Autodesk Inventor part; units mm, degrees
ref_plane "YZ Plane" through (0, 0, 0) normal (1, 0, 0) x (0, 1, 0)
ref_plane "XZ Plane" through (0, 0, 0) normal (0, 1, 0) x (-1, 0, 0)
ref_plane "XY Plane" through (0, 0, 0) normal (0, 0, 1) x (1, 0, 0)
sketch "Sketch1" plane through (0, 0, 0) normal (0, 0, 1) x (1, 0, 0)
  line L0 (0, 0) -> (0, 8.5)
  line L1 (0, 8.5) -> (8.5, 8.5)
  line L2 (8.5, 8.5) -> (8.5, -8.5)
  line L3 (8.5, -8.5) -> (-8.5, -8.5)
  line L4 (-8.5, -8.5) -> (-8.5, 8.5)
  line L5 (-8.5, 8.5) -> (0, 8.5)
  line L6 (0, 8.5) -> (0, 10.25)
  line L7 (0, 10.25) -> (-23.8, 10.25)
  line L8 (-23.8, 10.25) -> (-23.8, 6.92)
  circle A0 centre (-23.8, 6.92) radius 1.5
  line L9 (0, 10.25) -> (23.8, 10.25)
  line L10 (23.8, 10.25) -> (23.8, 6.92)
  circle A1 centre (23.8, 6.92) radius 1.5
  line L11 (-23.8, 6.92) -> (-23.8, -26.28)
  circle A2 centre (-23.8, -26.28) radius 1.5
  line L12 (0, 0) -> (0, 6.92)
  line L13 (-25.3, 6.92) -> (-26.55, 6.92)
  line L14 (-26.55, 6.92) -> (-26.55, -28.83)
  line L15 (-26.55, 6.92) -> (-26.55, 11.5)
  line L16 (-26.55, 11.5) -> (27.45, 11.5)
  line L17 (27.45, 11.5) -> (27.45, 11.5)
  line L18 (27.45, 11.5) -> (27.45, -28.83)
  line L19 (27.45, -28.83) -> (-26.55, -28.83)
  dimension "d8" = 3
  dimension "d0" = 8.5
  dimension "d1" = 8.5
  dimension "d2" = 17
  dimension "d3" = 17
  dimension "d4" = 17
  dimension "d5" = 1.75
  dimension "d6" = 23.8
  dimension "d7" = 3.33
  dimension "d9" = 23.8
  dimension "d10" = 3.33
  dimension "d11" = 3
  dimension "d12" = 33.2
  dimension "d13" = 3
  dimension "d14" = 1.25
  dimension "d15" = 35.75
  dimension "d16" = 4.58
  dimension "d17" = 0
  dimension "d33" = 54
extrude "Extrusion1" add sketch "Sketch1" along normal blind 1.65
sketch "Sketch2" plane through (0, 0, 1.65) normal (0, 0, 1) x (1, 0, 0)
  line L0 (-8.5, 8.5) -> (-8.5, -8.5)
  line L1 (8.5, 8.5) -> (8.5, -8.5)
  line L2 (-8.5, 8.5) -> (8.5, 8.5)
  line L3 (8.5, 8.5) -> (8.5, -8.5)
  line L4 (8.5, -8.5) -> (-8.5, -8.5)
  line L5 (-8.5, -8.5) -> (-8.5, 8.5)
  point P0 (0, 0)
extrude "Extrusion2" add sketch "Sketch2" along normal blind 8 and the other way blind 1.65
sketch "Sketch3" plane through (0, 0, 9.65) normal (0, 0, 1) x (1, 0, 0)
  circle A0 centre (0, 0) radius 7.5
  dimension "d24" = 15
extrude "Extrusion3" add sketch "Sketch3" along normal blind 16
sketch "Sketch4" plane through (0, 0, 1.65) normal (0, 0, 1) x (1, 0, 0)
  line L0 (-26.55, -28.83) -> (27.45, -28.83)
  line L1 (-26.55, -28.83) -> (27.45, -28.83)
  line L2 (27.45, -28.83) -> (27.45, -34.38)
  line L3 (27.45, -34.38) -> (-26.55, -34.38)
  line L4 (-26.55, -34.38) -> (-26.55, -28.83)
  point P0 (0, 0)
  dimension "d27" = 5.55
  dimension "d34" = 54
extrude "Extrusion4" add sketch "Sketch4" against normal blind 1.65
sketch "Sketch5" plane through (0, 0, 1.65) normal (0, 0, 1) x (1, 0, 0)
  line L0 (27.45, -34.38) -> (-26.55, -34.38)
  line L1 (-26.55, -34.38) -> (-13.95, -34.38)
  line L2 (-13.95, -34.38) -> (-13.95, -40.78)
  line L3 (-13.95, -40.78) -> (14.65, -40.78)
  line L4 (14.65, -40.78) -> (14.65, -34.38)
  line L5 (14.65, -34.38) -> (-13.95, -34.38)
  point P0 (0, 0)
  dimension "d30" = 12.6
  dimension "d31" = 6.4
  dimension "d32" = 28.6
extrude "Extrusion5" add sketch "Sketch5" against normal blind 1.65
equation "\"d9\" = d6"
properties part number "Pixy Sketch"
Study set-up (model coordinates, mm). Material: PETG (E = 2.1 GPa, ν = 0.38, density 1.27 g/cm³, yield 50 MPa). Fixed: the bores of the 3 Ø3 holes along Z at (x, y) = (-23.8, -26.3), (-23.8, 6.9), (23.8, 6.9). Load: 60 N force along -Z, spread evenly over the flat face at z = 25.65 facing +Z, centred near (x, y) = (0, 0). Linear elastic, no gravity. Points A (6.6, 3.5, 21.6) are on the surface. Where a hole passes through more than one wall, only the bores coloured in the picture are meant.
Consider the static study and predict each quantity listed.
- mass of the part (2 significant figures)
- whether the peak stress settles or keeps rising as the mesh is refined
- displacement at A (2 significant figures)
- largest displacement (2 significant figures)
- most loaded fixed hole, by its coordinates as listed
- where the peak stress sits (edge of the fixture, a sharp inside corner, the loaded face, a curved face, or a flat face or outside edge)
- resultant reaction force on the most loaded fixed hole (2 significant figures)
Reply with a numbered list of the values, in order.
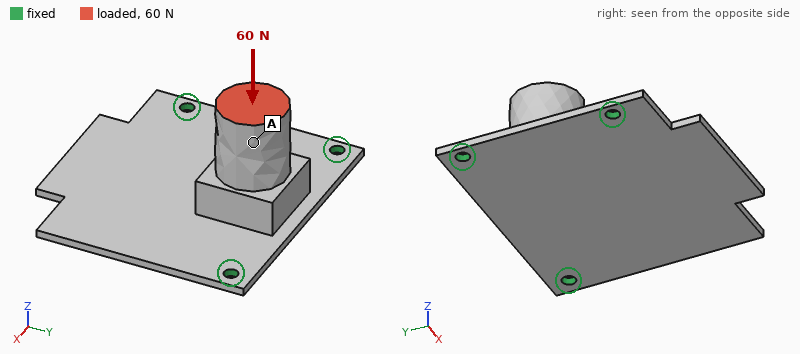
1. 12 g
2. keeps rising
3. 0.67 mm
4. 0.89 mm
5. (23.8, 6.9)
6. edge of the fixture
7. 31 N
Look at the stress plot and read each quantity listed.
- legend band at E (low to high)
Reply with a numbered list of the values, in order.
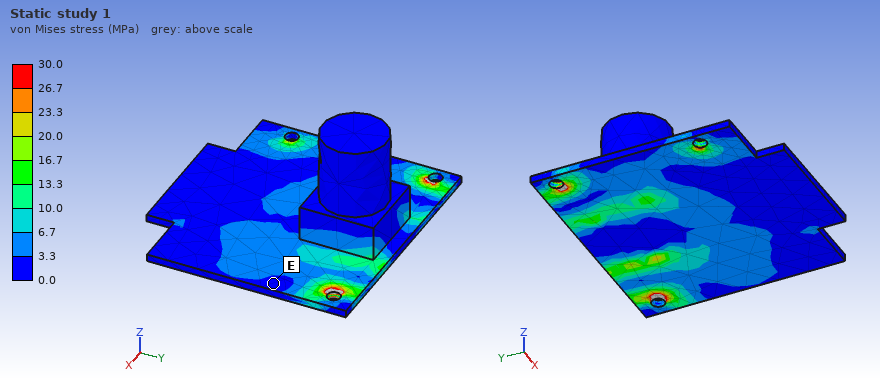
1. 0.0 to 3.3 MPa
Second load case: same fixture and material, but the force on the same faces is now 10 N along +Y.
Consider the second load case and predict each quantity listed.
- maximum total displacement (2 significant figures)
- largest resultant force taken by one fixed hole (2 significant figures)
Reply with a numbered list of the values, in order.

1. 0.80 mm
2. 7.6 N
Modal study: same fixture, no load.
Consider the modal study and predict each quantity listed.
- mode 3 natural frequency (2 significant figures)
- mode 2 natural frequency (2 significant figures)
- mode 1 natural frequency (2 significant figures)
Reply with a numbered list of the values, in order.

1. 590 Hz
2. 540 Hz
3. 280 Hz
